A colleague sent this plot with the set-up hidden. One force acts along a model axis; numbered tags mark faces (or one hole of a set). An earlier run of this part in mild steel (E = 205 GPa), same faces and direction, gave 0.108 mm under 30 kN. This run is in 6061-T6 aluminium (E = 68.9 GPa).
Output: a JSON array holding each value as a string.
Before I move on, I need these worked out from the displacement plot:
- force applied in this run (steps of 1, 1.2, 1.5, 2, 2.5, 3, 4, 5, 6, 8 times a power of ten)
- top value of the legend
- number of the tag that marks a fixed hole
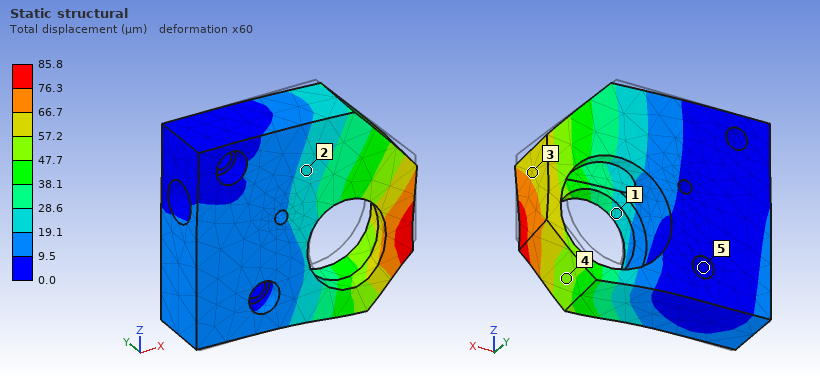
["8 kN", "85.8 µm", "5"]
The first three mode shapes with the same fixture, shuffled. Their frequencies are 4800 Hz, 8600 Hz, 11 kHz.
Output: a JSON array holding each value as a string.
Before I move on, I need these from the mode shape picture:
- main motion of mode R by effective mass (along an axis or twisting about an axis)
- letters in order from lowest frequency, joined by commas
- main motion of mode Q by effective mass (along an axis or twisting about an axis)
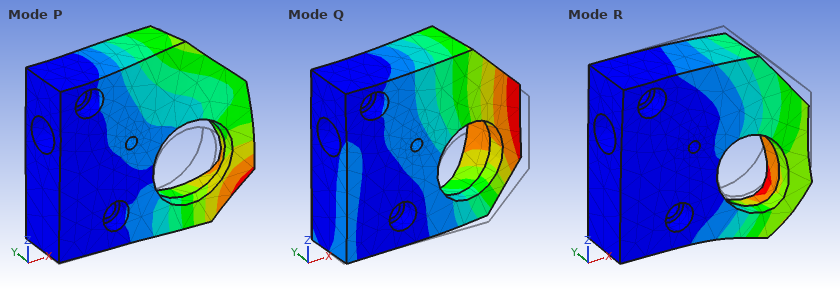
["along Z", "Q, R, P", "along Y"]
